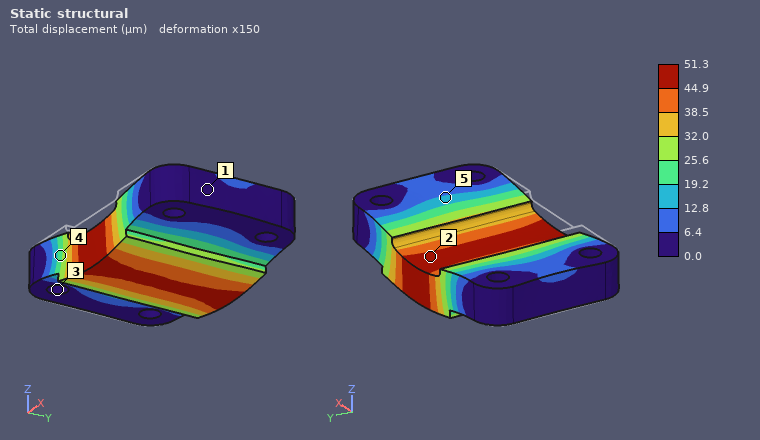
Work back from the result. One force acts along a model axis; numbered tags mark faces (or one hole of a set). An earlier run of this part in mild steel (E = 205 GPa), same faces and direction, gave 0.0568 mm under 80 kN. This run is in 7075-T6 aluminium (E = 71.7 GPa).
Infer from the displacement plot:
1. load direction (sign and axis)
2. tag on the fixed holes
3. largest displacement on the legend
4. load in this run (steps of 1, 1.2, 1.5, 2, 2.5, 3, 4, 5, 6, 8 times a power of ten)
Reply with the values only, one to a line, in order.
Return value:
-Z
3
51.3 µm
25 kN
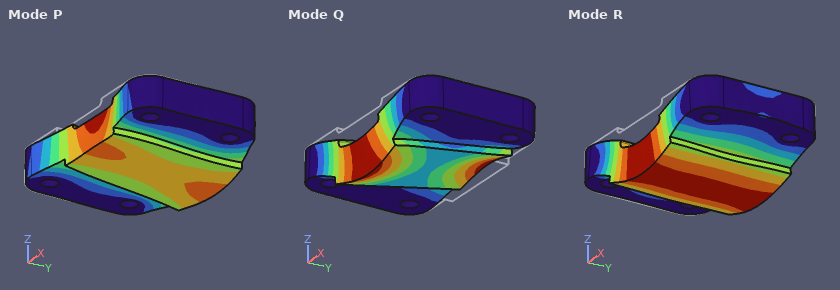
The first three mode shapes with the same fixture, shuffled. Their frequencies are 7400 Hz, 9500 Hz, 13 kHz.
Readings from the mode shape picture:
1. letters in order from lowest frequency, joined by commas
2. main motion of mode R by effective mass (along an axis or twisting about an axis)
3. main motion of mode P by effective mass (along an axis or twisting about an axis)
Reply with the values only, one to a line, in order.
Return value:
R, Q, P
along Z
along Y
